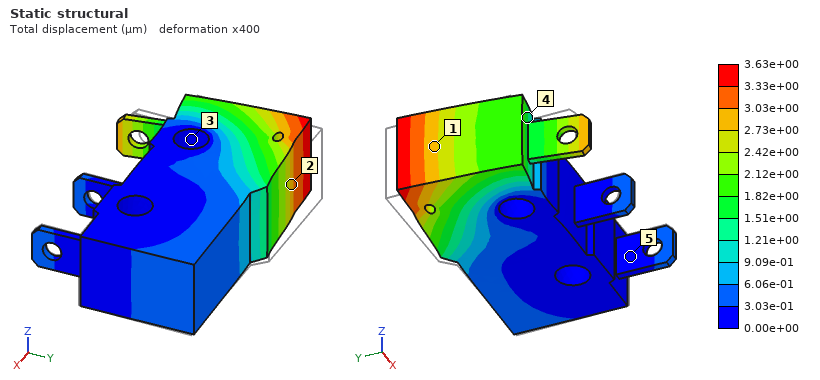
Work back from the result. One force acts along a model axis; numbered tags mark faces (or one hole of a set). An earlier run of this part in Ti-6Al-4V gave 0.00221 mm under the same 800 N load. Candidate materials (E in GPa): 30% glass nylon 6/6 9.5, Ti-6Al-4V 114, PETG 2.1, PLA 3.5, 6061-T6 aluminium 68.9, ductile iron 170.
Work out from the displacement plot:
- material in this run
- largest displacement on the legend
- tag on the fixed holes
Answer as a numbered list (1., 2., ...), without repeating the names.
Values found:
1. 6061-T6 aluminium
2. 3.63e+00 µm
3. 3
